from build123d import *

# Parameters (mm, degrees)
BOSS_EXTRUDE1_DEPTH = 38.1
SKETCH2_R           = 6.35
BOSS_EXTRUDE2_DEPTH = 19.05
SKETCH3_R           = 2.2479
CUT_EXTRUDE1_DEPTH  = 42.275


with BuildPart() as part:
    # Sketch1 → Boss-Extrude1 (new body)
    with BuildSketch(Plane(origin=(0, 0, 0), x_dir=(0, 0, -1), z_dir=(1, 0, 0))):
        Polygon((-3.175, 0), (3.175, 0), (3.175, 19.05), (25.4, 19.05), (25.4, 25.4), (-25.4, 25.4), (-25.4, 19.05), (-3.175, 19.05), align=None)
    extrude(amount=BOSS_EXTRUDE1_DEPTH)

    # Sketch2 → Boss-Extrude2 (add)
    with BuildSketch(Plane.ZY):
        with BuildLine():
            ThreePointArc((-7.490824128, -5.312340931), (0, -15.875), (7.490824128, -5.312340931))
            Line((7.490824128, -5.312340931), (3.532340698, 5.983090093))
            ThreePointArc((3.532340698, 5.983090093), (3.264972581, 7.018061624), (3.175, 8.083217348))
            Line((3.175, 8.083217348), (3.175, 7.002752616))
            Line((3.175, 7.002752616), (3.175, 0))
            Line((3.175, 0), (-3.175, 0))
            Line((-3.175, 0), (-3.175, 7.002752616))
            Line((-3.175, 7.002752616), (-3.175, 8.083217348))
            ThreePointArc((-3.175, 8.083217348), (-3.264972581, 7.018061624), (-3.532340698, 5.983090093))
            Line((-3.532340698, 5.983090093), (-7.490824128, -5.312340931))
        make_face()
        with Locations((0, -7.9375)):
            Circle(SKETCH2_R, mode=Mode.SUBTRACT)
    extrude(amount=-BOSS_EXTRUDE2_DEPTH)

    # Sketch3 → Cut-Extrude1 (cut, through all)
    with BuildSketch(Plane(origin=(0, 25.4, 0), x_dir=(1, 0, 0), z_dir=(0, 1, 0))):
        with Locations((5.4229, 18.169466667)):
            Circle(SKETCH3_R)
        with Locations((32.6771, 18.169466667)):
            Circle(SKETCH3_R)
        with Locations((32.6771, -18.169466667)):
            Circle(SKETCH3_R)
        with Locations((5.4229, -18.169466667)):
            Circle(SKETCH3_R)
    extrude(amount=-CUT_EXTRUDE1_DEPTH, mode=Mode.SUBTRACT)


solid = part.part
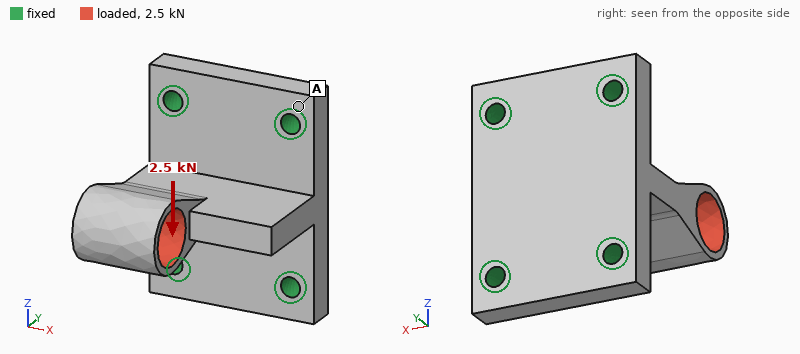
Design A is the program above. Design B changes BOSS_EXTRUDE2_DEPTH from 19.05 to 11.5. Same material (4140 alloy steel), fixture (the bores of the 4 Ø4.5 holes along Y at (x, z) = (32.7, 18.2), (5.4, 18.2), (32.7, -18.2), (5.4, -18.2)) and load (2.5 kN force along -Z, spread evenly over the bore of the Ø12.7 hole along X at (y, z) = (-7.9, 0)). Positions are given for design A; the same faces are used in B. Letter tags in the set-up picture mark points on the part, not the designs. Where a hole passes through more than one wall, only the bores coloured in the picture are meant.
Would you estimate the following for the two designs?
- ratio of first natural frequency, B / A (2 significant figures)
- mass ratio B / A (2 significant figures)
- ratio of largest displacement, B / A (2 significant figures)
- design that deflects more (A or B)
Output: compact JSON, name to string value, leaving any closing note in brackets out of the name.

{"ratio of first natural frequency, B / A": "1.1", "mass ratio B / A": "0.96", "ratio of largest displacement, B / A": "1.3", "design that deflects more": "B"}
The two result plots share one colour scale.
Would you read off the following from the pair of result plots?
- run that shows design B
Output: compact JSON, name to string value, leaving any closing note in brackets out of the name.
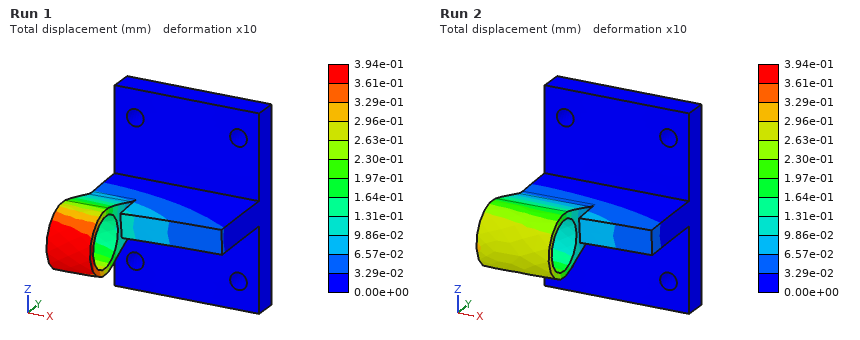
{"run that shows design B": "Run 1"}
